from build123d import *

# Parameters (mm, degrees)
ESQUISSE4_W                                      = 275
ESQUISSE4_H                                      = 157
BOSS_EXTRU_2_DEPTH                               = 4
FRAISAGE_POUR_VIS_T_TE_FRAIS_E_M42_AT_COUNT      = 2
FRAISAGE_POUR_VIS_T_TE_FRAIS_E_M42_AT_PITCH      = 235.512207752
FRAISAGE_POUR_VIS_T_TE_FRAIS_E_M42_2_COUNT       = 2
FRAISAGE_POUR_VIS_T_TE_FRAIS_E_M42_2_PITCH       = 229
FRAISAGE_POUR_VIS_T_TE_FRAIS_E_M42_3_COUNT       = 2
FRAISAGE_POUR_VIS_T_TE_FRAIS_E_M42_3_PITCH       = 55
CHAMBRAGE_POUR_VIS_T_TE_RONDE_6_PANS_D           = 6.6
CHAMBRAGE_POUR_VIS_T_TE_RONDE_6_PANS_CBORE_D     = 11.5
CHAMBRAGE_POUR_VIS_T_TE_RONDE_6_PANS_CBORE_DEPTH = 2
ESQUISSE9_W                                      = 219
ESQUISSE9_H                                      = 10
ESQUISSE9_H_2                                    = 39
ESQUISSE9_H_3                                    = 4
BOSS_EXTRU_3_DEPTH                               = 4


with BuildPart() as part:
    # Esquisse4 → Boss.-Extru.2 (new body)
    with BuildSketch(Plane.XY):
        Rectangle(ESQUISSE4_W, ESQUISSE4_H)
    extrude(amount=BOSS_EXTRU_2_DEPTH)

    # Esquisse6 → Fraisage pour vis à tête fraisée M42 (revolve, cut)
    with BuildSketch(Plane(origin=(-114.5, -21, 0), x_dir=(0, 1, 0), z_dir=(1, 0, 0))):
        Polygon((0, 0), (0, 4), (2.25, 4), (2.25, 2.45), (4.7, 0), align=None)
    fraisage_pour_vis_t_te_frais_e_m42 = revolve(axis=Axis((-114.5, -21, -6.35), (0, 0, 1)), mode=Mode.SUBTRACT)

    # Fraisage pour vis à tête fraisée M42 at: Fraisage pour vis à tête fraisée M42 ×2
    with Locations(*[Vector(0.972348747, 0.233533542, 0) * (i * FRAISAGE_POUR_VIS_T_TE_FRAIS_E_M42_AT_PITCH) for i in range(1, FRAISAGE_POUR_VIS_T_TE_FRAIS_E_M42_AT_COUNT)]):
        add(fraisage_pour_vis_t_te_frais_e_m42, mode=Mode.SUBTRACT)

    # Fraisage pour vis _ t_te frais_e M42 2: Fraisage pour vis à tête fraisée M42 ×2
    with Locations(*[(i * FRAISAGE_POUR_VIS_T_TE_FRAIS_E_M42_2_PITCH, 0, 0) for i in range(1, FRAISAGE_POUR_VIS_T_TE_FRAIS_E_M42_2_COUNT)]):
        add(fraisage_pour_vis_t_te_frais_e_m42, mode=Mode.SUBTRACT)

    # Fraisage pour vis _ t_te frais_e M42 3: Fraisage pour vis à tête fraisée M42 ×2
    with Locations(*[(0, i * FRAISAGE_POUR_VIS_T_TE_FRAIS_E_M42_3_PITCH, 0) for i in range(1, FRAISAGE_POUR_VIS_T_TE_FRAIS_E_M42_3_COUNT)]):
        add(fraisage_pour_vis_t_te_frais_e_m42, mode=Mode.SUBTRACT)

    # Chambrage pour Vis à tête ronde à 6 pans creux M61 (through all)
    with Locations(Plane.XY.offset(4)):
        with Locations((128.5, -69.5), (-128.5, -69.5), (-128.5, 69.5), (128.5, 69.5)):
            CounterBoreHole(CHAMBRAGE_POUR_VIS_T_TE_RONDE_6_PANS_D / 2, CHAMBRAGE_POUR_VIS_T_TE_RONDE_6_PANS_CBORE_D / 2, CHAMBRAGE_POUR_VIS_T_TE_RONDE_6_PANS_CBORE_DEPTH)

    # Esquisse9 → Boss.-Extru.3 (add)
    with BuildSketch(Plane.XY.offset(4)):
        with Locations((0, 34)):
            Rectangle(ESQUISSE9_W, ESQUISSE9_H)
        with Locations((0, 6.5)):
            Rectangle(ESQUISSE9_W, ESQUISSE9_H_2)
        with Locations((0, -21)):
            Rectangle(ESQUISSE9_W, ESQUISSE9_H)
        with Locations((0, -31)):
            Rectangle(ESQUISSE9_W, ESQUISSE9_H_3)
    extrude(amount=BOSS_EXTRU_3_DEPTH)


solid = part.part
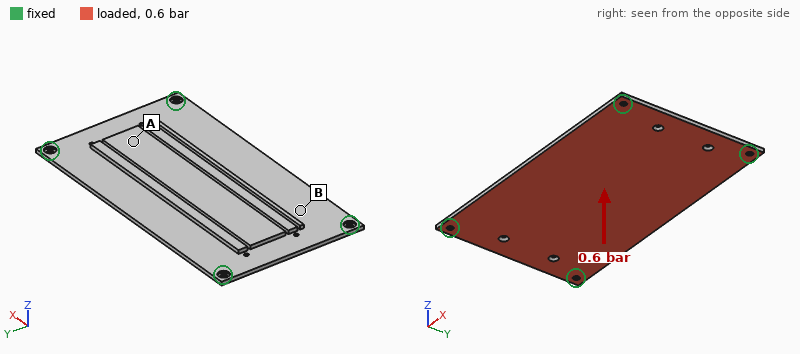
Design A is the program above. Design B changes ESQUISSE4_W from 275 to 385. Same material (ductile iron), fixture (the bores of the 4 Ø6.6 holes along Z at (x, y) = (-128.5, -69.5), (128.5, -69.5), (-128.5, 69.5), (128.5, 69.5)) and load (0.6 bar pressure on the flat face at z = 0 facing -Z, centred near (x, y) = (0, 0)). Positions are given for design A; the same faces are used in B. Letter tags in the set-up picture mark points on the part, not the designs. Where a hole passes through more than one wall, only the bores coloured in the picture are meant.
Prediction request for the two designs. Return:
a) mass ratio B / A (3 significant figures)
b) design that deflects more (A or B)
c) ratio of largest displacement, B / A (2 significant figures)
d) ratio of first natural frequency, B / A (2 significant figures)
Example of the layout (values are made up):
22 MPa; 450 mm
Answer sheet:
1.31; A; 0.86; 1.0
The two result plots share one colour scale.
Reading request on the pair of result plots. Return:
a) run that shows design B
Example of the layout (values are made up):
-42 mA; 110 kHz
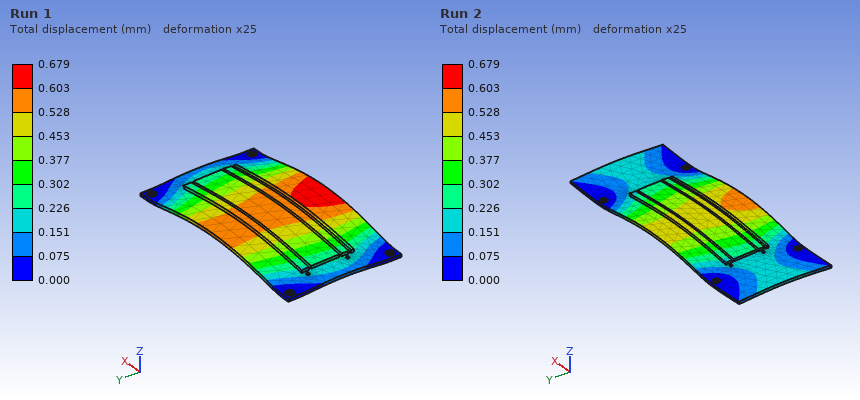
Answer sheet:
Run 2
